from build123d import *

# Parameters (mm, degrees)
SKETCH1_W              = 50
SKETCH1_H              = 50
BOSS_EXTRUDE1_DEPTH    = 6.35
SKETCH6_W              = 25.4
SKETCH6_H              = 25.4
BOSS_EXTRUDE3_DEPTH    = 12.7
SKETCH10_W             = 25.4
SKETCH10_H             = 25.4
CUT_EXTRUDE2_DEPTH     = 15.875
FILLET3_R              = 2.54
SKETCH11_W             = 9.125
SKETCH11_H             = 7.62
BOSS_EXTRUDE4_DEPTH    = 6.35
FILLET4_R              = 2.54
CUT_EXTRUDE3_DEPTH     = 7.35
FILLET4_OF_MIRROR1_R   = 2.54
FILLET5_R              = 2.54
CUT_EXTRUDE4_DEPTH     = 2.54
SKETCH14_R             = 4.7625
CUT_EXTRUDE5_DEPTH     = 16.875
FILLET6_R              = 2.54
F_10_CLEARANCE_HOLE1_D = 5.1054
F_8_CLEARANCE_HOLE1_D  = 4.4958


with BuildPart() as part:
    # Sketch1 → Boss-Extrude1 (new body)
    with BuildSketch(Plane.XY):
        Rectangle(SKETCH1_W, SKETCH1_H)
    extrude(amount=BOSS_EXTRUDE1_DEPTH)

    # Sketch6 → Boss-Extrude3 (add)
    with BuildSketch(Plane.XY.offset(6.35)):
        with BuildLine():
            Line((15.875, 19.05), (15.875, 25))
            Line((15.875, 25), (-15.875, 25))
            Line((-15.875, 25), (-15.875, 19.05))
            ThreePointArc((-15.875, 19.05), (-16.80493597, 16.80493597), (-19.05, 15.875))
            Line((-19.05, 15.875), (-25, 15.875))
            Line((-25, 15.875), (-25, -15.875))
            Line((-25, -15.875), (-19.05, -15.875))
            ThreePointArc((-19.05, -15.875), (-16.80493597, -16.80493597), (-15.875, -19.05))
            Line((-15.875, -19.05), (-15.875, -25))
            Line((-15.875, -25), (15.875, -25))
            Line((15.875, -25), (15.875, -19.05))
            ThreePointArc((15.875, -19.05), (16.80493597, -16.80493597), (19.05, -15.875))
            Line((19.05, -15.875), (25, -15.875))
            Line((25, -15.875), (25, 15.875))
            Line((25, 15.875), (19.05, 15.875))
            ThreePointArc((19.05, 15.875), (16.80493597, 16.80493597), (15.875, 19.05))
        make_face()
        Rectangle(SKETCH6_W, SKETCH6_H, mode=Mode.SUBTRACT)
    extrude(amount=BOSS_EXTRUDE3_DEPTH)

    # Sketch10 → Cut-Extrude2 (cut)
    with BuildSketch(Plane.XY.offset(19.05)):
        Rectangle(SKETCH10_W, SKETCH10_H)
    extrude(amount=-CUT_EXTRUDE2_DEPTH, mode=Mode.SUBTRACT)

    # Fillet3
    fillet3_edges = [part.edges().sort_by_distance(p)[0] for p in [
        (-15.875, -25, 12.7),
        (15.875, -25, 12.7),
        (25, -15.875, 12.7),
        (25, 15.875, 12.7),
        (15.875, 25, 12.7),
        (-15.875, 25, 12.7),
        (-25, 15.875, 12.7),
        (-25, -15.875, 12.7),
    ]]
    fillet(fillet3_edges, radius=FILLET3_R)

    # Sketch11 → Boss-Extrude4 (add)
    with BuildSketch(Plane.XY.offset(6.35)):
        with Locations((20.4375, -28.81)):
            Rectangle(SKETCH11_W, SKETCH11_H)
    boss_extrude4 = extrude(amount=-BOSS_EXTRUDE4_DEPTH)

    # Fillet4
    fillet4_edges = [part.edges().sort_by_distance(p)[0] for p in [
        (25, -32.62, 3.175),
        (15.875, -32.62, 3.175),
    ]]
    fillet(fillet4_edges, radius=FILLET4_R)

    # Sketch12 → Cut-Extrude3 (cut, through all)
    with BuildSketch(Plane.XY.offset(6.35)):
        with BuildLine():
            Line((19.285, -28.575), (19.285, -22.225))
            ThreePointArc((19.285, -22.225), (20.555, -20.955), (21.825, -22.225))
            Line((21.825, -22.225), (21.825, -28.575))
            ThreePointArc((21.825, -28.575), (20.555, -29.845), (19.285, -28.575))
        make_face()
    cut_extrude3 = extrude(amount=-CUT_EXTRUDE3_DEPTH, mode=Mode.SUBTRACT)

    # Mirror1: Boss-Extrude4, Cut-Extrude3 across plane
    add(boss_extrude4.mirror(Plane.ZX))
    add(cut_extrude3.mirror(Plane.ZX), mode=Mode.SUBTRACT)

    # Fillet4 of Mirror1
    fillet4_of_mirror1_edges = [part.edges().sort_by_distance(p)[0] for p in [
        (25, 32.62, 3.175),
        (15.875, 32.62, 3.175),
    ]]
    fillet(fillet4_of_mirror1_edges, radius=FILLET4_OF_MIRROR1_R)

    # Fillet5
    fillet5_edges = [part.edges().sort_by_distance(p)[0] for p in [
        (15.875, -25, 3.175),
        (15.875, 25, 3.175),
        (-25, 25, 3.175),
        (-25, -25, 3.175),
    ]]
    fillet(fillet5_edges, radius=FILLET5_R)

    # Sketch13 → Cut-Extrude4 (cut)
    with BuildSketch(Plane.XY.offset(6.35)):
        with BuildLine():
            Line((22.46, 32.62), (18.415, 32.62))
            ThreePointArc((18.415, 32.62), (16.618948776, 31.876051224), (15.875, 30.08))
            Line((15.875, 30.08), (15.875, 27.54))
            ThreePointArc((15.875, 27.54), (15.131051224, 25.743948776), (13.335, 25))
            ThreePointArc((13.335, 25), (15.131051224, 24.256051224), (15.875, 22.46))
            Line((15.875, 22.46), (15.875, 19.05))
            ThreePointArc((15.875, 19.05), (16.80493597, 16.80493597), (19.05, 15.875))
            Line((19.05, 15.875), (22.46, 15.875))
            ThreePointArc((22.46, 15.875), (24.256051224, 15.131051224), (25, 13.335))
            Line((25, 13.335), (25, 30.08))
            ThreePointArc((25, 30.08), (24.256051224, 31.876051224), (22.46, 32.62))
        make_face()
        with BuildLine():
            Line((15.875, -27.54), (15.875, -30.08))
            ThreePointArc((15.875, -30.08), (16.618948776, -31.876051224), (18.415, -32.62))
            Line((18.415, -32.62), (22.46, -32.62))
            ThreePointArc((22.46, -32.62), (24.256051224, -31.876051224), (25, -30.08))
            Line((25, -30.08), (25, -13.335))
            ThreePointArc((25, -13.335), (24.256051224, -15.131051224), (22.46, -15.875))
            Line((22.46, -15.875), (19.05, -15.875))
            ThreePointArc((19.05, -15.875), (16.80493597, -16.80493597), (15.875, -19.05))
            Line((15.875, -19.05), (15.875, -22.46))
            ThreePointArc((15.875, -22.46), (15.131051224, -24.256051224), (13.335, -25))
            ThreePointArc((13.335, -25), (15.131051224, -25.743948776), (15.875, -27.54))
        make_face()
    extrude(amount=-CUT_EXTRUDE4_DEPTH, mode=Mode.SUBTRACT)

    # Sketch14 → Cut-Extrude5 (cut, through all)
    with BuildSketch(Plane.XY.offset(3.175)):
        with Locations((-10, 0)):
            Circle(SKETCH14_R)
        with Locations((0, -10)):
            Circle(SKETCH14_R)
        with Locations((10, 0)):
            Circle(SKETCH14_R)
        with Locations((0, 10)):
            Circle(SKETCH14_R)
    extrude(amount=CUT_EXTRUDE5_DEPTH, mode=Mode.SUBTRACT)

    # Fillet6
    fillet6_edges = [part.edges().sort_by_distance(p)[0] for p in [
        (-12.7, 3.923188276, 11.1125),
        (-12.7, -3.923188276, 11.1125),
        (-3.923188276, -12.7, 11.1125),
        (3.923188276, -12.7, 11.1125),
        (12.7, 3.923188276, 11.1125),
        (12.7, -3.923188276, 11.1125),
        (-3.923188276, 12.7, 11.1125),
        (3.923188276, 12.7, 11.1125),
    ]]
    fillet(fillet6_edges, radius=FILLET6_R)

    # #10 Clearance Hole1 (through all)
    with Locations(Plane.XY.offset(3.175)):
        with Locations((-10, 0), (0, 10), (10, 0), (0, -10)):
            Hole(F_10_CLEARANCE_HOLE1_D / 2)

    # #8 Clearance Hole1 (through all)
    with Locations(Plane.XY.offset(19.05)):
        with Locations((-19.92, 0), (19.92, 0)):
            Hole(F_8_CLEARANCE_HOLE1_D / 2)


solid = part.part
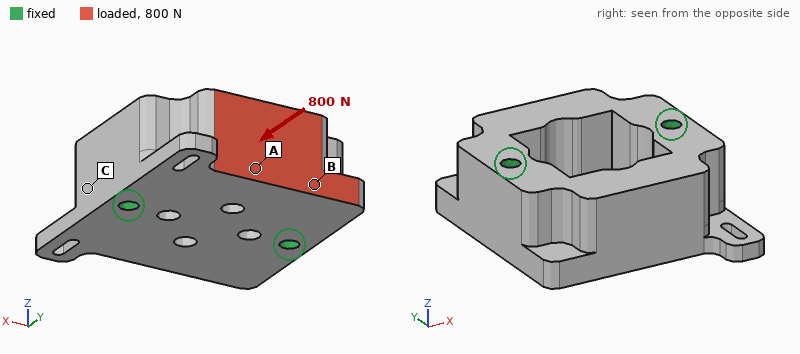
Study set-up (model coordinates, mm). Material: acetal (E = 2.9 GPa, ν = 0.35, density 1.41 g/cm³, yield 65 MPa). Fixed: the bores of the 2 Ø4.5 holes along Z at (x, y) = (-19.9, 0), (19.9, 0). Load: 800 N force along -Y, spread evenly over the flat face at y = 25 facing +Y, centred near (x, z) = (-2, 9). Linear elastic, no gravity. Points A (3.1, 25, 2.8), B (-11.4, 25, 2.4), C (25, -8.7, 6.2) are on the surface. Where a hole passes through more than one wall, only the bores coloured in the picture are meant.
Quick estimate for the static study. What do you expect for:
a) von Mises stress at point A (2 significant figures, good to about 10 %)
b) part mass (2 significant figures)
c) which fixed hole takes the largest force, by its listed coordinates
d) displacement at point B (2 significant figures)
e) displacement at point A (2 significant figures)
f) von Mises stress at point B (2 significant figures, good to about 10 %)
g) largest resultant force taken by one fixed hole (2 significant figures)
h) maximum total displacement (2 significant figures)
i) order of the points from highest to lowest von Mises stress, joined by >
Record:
2.4 MPa
44 g
(-19.9, 0)
21 µm
27 µm
1.3 MPa
460 N
48 µm
A > B > C
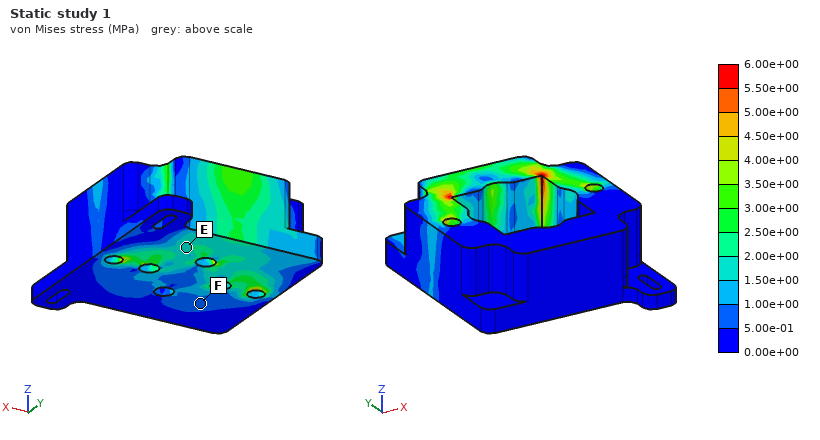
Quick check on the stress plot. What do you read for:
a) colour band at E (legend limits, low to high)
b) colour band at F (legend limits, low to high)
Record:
1.50e+00 to 2.00e+00 MPa
5.00e-01 to 1.00e+00 MPa
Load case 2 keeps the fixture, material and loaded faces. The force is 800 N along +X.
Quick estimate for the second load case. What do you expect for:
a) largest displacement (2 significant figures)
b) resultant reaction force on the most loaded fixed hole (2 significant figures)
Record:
71 µm
580 N
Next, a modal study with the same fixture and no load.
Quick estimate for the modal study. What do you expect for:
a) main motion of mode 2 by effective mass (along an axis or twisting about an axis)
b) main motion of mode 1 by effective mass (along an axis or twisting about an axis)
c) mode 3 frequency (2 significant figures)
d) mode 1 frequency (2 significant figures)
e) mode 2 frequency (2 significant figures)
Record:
along Z
twisting about X
4600 Hz
3500 Hz
3800 Hz
